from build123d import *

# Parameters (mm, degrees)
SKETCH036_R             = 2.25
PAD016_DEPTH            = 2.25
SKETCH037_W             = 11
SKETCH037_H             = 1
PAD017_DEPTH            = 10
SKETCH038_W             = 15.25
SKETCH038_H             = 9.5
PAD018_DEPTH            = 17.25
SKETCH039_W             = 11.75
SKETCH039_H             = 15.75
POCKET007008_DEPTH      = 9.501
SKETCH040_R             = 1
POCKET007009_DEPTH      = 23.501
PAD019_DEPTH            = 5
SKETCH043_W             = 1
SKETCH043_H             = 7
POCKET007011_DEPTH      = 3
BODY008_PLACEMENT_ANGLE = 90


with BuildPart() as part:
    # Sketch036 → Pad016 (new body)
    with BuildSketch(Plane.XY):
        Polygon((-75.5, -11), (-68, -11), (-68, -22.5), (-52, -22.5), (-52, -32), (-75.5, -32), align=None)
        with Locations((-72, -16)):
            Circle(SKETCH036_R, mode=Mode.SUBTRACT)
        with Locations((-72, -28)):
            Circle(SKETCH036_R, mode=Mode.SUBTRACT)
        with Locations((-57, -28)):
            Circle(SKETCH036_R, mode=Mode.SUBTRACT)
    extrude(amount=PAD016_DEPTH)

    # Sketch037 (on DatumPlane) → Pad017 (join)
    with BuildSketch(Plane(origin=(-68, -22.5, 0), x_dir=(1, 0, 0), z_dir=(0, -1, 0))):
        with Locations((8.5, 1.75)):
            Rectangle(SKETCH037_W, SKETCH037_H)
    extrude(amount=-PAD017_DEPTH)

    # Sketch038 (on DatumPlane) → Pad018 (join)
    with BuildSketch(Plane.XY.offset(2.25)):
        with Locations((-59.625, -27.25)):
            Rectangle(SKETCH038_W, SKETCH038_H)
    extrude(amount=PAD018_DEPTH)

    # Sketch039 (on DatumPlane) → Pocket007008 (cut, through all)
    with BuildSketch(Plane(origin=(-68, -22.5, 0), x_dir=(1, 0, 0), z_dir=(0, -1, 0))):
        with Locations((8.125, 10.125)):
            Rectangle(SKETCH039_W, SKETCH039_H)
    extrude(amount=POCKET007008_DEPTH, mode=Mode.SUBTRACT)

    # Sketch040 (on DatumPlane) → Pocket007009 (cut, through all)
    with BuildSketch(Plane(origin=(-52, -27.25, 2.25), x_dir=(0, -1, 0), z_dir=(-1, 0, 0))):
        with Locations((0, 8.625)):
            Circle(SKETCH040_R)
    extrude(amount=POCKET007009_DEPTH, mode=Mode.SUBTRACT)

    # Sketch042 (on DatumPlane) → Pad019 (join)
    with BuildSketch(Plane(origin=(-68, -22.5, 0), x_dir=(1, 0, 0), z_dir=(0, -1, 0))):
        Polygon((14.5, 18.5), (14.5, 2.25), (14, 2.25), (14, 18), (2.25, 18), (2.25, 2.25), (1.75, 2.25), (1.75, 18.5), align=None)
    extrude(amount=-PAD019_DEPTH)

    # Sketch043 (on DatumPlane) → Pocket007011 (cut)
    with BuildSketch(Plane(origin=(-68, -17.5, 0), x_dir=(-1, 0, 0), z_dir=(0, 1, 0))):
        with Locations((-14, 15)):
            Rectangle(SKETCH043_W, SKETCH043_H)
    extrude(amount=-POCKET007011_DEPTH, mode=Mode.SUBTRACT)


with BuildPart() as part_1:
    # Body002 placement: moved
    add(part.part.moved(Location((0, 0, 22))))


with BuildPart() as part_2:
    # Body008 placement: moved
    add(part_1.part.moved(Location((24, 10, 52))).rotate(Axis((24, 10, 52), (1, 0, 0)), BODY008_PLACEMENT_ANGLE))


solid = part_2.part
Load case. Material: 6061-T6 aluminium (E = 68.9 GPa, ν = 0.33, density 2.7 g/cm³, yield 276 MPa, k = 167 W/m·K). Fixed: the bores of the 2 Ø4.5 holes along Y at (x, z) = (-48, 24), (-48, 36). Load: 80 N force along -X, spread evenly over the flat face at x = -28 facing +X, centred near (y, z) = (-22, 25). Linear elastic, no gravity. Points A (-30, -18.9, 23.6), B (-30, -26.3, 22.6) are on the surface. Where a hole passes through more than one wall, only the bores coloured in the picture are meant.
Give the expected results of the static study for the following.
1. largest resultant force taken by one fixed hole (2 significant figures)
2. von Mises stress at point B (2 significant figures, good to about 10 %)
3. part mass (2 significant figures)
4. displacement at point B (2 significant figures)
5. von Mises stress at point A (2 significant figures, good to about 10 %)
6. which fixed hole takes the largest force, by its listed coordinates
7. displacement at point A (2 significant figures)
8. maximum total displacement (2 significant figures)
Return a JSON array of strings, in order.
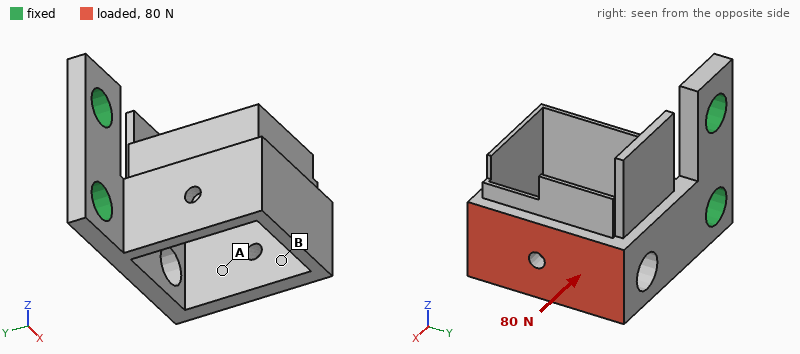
["74 N", "22 MPa", "4.1 g", "0.16 mm", "9.3 MPa", "(-48, 24)", "0.11 mm", "0.20 mm"]
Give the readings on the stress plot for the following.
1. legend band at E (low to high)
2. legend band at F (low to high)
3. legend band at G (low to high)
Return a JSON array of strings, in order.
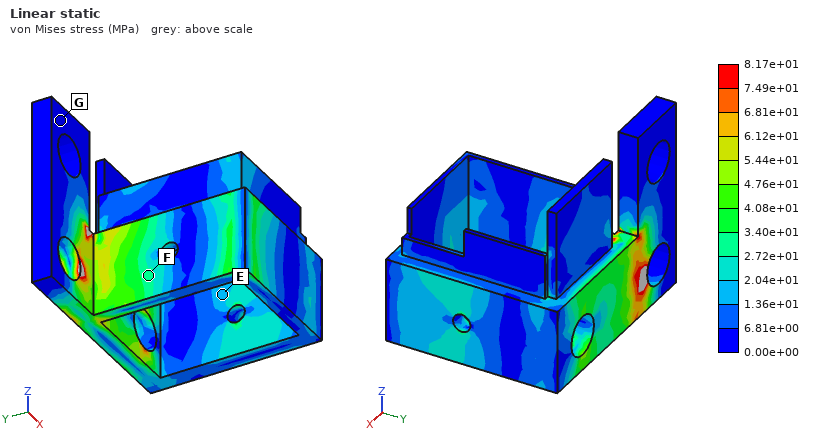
["1.36e+01 to 2.04e+01 MPa", "2.72e+01 to 3.40e+01 MPa", "0.00e+00 to 6.81e+00 MPa"]
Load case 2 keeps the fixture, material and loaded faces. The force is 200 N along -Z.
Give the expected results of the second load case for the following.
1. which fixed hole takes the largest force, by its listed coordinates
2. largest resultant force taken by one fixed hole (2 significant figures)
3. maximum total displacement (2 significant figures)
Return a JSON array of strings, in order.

["(-48, 36)", "260 N", "0.31 mm"]
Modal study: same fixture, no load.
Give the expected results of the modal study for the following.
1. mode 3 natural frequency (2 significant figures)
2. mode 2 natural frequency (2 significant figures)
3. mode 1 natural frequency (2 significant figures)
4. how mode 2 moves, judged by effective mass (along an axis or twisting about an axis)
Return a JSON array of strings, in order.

["6100 Hz", "3500 Hz", "1800 Hz", "along Z"]
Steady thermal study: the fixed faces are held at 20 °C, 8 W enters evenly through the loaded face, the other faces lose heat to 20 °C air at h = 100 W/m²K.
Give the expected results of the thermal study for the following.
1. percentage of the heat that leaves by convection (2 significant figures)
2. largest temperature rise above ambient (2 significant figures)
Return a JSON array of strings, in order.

["37 %", "28 K"]
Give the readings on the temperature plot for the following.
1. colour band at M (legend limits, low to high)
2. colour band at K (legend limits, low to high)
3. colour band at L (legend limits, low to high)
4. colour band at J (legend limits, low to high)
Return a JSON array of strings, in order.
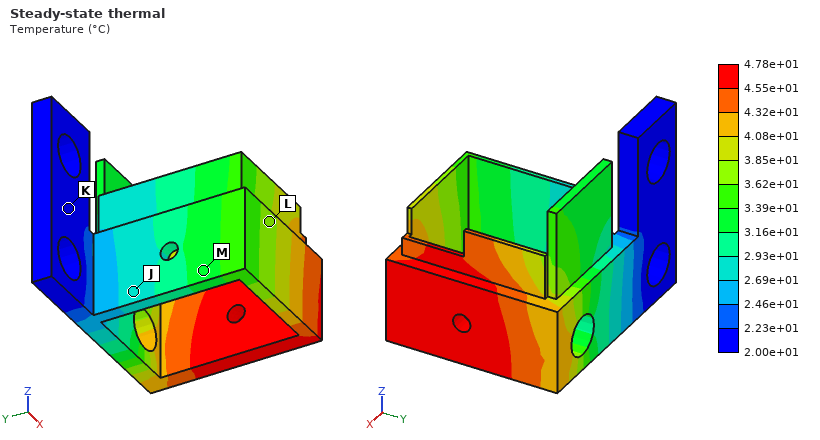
["3.16e+01 to 3.39e+01 °C", "2.00e+01 to 2.23e+01 °C", "3.62e+01 to 3.85e+01 °C", "2.69e+01 to 2.93e+01 °C"]
